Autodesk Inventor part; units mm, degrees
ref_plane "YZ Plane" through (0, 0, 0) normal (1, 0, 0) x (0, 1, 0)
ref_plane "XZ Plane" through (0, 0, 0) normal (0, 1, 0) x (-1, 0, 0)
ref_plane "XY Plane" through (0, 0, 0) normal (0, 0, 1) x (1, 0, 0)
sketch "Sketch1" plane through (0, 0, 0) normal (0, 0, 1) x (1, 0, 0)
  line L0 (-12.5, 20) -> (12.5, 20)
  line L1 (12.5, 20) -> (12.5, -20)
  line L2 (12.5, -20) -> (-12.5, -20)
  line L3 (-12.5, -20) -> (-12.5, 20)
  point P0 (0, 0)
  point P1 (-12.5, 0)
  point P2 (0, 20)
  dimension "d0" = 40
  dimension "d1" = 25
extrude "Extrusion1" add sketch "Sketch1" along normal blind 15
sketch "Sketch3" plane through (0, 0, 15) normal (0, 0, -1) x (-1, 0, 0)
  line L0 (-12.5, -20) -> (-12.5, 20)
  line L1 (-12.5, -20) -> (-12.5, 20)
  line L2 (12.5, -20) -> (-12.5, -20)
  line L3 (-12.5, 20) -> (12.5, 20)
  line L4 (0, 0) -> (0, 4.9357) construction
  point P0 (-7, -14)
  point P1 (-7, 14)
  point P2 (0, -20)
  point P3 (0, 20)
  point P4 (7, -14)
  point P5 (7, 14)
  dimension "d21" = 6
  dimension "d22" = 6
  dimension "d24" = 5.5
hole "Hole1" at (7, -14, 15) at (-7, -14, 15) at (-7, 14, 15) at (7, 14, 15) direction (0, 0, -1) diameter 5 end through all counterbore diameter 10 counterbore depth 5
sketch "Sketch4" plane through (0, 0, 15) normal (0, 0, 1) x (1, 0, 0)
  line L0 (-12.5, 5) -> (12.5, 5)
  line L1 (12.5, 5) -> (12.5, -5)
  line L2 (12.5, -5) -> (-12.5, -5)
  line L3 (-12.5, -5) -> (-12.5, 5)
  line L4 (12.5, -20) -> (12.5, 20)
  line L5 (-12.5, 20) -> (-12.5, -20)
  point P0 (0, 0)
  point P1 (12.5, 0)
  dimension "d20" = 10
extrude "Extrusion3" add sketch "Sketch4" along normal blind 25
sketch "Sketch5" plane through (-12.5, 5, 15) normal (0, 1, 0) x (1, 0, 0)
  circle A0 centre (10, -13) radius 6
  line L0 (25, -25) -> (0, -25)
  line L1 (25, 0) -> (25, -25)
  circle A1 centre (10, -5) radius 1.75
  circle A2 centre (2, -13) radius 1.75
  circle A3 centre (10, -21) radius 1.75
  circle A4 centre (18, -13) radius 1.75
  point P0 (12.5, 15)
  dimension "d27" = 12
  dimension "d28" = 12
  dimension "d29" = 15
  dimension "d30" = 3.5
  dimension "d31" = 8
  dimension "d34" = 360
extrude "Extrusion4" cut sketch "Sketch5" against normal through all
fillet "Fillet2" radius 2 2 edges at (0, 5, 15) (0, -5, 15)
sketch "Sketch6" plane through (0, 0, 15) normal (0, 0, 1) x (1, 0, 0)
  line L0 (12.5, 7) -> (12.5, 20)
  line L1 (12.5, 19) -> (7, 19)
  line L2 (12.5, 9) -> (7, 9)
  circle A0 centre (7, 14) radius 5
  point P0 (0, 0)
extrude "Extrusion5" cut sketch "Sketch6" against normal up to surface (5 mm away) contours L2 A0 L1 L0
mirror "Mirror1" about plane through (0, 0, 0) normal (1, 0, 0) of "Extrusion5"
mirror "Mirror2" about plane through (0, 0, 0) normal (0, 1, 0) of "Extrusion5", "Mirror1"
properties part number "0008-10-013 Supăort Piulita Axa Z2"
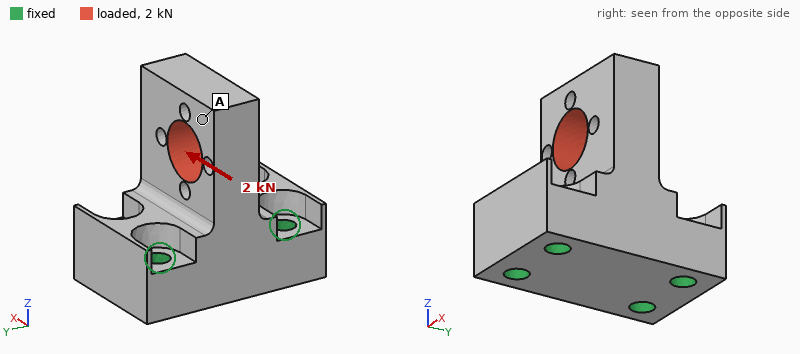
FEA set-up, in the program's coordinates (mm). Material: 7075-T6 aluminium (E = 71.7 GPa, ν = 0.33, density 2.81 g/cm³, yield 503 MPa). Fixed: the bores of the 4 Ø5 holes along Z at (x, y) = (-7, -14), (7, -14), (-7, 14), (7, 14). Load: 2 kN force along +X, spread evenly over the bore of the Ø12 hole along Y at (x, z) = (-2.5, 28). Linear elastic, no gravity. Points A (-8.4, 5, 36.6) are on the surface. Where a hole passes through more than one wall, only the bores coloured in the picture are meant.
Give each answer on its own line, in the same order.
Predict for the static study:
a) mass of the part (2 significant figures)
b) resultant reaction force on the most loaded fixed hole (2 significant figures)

48 g
1.4 kN
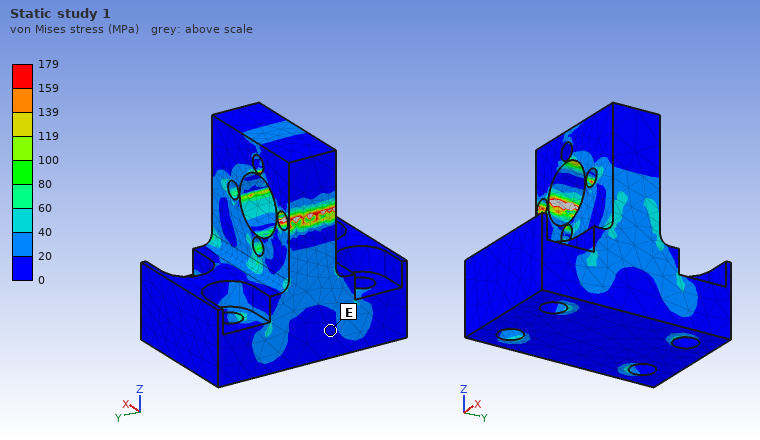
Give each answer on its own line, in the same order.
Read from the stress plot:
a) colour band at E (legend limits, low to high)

0 to 20 MPa
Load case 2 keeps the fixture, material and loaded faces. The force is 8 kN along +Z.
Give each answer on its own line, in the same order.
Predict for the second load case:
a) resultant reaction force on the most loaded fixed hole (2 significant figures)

2.7 kN
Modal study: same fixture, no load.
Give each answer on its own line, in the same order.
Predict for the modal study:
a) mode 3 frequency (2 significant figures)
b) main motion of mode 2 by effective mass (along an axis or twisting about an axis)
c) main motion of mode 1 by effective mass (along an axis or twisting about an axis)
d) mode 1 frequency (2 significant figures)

16 kHz
along X
along Y
8600 Hz
